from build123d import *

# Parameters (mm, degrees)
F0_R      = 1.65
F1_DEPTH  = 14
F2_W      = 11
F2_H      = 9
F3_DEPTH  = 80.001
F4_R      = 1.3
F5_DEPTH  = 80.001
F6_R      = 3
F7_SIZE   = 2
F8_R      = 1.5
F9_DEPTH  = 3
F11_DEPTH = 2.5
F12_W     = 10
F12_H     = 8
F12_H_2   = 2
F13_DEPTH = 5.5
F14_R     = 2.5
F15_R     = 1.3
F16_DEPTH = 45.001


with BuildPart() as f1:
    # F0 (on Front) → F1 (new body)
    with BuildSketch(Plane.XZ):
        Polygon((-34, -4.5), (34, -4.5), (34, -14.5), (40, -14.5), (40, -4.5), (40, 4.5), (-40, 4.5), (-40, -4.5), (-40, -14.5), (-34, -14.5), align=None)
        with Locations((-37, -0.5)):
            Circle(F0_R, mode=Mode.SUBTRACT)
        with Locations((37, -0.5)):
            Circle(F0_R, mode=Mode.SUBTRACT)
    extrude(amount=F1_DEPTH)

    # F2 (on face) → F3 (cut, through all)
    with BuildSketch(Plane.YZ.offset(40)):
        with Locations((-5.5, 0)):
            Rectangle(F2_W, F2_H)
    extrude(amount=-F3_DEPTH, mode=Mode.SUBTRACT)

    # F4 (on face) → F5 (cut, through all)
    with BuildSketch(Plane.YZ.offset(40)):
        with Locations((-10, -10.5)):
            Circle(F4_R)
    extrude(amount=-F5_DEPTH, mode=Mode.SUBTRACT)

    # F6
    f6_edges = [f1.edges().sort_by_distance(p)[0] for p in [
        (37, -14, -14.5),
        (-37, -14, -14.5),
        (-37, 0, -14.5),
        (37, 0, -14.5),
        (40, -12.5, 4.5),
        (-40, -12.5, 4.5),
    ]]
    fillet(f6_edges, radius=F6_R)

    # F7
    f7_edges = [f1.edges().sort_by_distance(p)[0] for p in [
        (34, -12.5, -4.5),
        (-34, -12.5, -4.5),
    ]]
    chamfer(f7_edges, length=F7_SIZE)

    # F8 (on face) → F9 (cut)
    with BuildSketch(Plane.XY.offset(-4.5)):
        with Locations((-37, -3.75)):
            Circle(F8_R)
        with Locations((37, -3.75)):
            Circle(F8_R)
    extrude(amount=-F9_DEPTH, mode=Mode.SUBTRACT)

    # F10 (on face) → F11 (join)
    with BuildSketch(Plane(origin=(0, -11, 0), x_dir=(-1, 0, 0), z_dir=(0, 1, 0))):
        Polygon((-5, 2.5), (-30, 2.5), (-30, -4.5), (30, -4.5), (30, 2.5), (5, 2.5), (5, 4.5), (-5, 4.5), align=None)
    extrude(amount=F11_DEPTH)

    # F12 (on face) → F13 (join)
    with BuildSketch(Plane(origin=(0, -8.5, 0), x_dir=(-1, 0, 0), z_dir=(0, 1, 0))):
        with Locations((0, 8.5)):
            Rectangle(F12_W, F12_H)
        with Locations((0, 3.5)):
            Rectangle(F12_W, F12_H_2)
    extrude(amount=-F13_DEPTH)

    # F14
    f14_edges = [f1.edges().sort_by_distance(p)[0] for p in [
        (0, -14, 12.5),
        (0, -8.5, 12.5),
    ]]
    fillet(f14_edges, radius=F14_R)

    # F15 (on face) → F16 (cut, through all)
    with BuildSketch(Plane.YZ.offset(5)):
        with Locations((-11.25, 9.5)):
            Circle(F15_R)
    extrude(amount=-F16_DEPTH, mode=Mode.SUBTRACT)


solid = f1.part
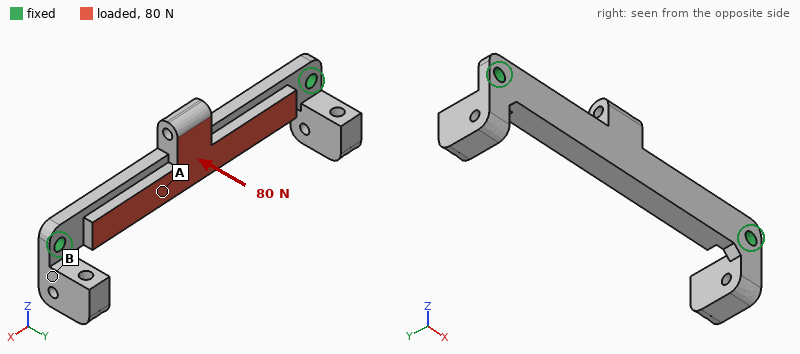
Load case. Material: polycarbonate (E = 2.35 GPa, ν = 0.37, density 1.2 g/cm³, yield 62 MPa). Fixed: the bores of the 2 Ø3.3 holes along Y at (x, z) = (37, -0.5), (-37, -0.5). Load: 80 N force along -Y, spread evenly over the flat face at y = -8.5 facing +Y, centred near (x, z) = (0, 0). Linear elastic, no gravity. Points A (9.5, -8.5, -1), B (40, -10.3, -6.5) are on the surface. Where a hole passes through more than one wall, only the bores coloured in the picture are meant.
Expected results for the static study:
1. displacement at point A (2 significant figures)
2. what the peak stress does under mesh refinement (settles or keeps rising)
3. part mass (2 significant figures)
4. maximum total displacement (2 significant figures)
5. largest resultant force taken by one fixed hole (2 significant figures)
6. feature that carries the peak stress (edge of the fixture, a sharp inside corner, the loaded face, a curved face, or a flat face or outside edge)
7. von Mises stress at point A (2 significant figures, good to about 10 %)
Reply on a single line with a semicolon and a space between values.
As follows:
0.65 mm; keeps rising; 6.1 g; 0.84 mm; 87 N; edge of the fixture; 12 MPa
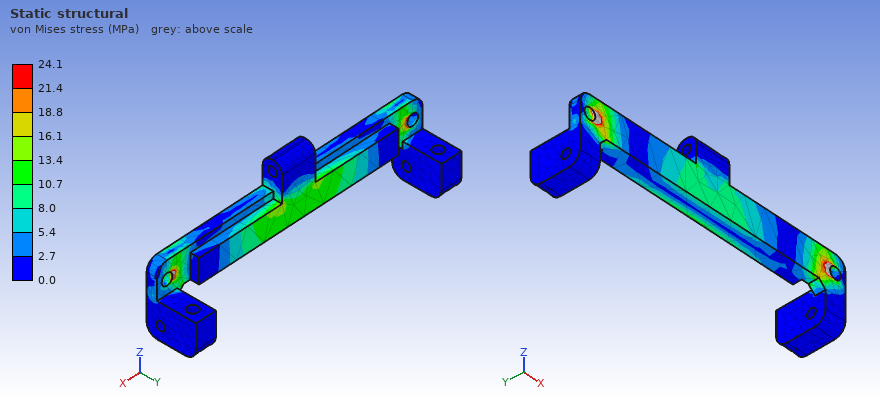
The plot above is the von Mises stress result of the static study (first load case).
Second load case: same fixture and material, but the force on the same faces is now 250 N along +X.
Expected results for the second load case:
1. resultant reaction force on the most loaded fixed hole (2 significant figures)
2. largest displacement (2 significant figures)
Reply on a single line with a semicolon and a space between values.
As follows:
130 N; 68 µm
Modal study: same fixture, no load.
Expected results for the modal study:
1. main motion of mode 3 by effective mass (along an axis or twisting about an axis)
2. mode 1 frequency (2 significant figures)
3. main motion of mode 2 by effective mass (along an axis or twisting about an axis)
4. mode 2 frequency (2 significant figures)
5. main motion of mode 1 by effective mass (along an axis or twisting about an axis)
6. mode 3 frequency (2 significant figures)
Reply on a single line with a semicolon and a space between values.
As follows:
along Y; 930 Hz; along Z; 1500 Hz; along Y; 1600 Hz
